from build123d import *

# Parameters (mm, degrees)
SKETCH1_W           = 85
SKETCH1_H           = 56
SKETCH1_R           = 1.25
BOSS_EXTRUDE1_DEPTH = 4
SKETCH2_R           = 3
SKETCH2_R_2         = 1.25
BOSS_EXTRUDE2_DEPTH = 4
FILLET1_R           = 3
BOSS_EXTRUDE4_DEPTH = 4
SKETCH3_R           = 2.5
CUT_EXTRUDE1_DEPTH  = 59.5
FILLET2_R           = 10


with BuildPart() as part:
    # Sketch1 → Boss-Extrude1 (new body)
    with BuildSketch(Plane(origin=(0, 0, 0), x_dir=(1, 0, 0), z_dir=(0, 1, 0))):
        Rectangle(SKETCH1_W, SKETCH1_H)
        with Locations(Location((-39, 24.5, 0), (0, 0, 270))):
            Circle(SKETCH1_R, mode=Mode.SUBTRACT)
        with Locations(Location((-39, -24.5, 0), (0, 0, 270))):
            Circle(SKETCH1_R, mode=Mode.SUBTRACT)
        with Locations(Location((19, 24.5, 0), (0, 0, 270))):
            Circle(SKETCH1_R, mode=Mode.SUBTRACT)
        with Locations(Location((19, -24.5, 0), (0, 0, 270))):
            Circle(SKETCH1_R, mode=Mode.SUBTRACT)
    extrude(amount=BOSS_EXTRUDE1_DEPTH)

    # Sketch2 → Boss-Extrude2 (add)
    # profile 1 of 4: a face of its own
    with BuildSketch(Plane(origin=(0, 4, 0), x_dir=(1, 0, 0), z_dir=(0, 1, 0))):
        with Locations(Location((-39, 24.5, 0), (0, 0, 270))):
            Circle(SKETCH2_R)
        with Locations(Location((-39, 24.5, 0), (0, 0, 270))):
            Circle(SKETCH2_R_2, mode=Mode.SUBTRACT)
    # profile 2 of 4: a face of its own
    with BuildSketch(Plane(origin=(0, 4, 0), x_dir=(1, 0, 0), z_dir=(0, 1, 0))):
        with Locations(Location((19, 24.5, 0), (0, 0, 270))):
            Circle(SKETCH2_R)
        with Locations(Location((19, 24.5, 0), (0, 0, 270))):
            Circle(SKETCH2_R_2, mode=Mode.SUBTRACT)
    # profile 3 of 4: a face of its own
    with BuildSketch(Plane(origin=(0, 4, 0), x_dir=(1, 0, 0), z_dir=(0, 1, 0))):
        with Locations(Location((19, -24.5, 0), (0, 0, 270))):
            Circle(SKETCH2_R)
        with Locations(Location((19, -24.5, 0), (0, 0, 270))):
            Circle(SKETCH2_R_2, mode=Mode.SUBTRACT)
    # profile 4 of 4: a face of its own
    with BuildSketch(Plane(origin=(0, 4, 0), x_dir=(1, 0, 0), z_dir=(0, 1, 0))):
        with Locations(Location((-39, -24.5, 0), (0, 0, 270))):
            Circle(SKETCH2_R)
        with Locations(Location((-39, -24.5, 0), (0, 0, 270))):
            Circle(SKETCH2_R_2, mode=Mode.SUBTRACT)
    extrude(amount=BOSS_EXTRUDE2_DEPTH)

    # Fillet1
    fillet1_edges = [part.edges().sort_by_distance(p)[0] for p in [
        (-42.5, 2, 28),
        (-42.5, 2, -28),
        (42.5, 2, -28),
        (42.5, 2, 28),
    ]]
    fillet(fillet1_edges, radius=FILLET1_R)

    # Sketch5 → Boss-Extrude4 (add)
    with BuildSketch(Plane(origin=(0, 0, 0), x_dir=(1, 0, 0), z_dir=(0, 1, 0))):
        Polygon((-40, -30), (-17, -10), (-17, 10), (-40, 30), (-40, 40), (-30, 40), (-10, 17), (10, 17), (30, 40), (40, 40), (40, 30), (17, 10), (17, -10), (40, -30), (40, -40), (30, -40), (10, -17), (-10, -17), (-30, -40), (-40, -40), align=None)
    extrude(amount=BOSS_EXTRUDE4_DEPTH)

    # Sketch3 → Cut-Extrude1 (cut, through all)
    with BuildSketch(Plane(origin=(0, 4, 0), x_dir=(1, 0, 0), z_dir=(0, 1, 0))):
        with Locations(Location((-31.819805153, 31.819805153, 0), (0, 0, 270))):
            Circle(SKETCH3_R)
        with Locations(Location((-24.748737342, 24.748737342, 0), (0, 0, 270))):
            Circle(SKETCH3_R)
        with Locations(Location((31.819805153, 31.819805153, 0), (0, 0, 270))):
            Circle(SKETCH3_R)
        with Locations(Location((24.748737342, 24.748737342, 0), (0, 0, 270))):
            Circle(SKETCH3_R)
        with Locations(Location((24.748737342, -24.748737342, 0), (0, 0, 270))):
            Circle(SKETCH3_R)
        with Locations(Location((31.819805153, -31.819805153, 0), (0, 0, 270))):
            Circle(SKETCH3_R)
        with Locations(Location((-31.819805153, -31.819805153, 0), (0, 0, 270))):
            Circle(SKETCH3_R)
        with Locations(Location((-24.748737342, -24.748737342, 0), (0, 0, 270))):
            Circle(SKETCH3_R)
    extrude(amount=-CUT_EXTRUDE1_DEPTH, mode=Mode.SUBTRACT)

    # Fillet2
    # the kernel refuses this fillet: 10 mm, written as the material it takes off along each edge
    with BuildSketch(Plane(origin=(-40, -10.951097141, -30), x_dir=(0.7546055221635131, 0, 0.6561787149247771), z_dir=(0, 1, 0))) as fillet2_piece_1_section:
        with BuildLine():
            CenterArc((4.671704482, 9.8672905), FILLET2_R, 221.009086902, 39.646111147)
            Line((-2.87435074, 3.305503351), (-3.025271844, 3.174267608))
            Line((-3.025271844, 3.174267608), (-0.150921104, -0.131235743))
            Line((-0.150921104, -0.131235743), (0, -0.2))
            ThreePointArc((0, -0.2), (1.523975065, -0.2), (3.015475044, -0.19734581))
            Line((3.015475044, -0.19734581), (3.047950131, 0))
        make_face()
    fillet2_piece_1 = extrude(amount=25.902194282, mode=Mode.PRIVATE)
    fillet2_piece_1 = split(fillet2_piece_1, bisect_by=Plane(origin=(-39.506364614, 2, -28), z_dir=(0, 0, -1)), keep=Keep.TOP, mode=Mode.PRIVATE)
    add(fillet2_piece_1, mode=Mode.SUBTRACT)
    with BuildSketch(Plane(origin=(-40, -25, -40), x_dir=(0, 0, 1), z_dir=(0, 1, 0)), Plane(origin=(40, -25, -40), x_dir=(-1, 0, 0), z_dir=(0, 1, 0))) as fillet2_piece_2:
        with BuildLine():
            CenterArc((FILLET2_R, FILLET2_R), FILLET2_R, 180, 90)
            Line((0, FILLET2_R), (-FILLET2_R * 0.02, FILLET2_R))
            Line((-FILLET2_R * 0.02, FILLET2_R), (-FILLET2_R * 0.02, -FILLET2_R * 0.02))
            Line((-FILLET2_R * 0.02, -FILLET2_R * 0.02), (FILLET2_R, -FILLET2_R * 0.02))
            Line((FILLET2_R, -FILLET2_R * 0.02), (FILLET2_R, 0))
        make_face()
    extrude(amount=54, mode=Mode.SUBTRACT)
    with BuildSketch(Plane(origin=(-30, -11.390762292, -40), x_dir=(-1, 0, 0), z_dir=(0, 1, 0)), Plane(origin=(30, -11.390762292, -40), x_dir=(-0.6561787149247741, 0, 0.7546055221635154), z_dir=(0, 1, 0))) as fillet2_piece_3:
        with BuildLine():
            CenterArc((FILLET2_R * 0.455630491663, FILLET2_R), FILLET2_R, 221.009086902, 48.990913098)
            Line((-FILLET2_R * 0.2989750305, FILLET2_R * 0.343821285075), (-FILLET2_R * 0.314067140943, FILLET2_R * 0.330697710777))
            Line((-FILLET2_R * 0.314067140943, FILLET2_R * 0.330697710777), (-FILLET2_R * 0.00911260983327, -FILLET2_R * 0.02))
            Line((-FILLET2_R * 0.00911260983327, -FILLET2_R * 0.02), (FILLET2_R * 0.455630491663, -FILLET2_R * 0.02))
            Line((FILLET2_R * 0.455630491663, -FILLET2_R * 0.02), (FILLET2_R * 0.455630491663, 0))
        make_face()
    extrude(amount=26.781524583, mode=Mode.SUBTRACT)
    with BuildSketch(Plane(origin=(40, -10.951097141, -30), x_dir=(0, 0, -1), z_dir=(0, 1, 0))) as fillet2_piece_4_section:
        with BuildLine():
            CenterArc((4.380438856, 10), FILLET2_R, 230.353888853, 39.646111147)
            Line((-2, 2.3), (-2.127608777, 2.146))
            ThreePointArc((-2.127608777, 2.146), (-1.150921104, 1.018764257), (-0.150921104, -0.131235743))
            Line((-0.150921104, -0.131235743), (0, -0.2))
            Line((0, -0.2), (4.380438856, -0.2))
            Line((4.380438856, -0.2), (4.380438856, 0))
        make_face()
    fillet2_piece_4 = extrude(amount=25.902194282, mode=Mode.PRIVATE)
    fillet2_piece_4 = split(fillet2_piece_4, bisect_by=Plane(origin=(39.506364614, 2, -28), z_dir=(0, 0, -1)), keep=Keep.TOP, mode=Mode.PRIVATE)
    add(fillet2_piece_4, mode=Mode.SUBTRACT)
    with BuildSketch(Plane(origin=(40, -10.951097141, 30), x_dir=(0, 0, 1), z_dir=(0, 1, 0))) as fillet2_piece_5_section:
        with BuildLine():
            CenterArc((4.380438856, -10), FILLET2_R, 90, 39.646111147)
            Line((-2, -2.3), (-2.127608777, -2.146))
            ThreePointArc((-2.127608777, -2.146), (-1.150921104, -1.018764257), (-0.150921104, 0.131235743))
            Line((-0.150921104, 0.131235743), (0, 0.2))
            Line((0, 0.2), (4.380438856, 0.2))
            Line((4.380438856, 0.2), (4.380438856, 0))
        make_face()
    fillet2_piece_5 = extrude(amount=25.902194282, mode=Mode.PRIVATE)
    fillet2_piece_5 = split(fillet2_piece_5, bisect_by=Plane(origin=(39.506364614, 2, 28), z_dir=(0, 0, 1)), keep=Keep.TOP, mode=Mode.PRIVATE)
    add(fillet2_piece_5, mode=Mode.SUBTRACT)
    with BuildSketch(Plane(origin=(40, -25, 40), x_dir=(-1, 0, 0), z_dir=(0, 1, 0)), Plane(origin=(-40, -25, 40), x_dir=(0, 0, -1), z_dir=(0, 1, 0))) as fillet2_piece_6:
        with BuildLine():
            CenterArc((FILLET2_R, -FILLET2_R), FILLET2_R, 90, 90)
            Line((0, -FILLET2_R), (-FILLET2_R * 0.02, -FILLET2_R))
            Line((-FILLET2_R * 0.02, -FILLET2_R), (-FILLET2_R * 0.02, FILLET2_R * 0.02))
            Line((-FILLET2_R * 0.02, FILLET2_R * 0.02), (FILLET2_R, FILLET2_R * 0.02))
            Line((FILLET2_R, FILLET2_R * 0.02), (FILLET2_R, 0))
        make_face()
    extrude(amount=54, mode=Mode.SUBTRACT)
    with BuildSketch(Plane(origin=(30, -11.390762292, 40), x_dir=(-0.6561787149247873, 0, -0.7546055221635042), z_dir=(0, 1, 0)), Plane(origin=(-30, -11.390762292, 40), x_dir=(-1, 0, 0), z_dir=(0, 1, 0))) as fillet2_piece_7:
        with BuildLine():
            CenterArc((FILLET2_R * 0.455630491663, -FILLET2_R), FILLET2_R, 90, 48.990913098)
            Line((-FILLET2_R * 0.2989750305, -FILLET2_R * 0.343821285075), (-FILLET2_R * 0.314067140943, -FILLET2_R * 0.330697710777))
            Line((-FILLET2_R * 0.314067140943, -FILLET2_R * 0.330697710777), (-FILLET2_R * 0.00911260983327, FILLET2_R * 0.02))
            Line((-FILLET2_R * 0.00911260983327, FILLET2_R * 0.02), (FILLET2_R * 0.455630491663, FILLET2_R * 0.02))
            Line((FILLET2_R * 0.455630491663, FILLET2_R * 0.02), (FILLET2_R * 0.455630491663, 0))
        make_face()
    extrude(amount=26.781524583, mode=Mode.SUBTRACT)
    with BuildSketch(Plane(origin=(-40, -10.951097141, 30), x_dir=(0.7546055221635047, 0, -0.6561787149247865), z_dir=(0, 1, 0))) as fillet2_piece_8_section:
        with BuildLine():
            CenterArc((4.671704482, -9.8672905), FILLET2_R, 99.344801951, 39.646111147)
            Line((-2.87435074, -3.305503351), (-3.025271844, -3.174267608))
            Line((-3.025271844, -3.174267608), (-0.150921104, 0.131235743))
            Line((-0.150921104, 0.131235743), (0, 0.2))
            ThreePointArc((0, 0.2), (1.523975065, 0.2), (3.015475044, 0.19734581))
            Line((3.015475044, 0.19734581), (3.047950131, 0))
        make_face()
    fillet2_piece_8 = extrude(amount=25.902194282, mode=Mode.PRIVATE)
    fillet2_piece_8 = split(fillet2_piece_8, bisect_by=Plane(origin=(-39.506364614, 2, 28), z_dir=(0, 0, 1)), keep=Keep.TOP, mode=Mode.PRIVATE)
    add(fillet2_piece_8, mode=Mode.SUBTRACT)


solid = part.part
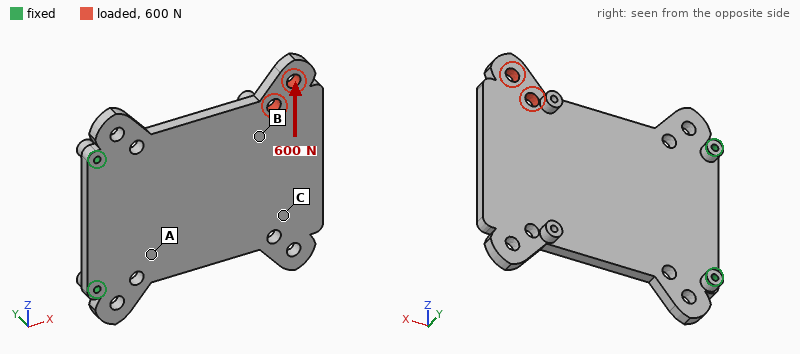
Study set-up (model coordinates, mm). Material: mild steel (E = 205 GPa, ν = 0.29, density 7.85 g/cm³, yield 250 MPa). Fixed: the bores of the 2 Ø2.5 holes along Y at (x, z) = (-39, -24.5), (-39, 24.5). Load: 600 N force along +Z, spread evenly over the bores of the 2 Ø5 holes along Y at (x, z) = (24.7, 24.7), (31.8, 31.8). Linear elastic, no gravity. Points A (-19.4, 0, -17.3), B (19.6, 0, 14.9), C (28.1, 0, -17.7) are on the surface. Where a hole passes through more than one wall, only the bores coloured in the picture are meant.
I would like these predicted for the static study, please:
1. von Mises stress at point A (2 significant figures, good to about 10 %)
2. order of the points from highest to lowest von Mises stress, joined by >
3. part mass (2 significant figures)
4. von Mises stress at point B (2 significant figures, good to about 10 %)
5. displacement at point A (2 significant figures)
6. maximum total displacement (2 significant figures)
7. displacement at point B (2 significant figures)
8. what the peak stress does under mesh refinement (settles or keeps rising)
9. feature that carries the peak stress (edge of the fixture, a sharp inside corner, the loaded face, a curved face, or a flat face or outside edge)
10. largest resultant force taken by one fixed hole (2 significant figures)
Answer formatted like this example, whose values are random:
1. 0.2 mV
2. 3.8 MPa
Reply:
1. 10 MPa
2. A > B > C
3. 170 g
4. 7.3 MPa
5. 2.1 µm
6. 12 µm
7. 7.8 µm
8. keeps rising
9. edge of the fixture
10. 870 N
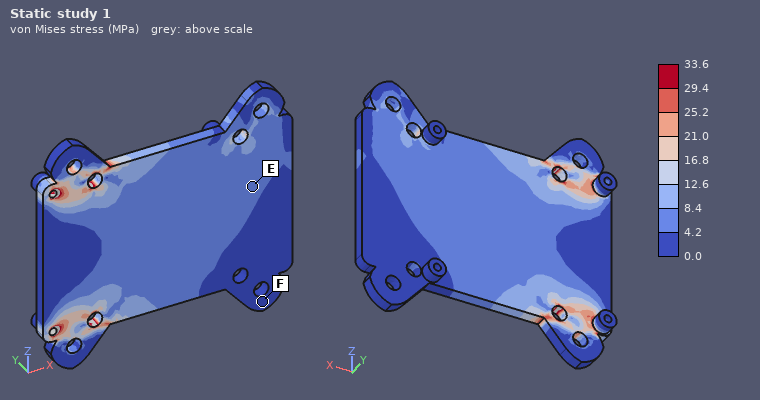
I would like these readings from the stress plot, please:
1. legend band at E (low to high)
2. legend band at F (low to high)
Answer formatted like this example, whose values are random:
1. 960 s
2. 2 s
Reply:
1. 4.2 to 8.4 MPa
2. 0.0 to 4.2 MPa
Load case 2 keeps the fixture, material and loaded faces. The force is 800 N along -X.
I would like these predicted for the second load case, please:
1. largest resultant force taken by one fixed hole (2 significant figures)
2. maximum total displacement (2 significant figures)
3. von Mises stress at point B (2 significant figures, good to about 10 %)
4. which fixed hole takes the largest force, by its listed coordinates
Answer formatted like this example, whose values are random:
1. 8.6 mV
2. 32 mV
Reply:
1. 870 N
2. 11 µm
3. 6.5 MPa
4. (-39, 24.5)
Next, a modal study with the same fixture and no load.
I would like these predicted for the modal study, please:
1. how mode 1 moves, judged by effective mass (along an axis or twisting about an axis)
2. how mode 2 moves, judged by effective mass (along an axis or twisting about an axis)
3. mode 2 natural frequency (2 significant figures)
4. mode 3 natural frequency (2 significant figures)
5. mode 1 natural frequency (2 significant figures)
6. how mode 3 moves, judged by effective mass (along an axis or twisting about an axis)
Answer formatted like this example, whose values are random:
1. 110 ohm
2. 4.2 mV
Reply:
1. along Y
2. twisting about X
3. 1300 Hz
4. 2800 Hz
5. 410 Hz
6. along Y
